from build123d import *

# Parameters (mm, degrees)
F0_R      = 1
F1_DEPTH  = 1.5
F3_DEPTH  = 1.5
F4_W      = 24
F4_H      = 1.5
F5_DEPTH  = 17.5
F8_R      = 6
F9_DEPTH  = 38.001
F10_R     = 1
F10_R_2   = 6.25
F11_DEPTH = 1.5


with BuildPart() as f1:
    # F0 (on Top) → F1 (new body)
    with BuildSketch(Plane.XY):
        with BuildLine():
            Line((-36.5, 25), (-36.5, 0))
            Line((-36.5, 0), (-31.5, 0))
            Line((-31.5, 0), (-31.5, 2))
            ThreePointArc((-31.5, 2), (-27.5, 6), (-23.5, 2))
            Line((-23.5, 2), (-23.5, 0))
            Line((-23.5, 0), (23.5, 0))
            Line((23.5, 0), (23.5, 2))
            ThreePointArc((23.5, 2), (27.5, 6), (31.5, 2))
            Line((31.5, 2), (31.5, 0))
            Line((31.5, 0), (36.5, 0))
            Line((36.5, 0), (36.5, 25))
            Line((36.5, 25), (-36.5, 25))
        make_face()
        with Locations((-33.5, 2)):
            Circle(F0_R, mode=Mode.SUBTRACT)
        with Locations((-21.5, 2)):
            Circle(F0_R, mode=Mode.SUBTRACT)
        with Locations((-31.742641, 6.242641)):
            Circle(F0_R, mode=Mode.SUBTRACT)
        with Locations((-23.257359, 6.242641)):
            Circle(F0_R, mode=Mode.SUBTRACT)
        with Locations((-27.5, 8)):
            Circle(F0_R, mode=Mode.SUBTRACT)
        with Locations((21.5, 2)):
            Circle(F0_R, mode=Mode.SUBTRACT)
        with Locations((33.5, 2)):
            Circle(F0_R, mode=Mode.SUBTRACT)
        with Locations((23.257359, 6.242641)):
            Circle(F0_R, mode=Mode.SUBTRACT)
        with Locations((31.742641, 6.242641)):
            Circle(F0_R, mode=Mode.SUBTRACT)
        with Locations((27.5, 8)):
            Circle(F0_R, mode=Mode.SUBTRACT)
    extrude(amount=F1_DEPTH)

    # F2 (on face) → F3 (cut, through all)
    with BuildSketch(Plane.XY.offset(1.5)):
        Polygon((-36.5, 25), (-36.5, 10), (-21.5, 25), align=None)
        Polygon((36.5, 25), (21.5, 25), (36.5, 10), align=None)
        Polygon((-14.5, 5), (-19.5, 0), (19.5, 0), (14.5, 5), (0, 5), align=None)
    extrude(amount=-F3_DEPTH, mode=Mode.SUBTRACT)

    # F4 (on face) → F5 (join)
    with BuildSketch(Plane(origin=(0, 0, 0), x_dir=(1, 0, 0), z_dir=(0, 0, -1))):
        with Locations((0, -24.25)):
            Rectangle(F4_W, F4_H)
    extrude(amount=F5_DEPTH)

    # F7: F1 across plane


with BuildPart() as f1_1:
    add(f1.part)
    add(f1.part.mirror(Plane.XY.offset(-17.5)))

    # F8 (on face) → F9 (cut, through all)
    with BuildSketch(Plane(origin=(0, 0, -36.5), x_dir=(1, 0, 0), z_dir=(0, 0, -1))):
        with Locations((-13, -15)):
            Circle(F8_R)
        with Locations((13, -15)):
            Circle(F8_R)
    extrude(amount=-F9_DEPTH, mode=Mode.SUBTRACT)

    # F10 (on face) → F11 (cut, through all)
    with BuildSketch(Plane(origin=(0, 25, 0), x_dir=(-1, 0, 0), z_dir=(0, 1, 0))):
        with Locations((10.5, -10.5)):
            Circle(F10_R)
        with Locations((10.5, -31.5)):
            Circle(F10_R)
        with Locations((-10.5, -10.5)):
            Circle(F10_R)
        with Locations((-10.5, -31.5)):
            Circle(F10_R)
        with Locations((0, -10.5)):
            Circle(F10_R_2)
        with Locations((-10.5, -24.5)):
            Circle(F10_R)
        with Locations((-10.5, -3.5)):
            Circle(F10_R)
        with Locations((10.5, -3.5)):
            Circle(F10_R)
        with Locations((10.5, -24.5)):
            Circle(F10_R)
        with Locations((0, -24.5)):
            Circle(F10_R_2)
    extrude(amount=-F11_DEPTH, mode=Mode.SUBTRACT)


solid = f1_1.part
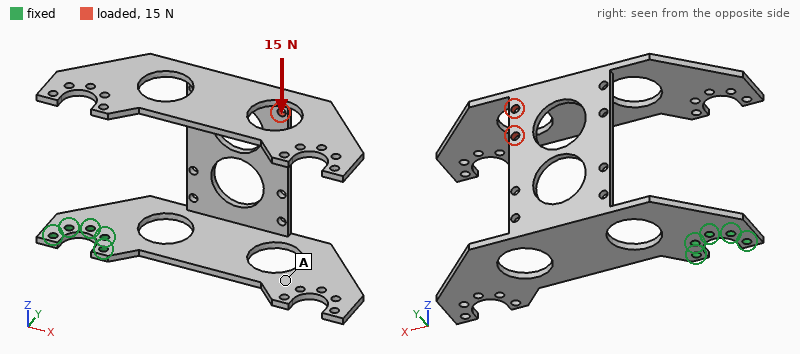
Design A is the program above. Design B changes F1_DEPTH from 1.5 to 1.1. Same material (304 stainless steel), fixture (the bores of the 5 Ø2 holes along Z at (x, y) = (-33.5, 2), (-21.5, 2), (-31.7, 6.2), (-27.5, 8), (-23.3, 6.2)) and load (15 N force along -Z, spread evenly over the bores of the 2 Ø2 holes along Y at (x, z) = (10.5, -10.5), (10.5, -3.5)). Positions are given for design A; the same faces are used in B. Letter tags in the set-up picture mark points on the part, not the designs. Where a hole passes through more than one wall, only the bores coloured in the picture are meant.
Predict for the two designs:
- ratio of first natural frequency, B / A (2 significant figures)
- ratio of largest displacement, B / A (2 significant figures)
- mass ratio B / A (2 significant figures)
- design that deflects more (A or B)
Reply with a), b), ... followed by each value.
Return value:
a) 0.74
b) 2.4
c) 0.79
d) B
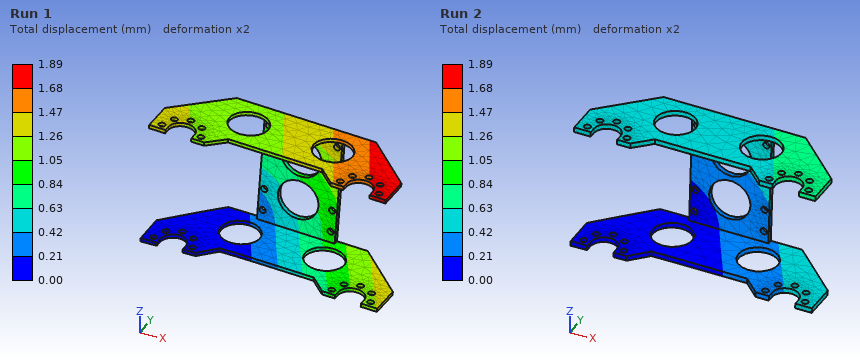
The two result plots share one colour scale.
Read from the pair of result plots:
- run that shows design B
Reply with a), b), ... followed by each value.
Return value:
a) Run 1
